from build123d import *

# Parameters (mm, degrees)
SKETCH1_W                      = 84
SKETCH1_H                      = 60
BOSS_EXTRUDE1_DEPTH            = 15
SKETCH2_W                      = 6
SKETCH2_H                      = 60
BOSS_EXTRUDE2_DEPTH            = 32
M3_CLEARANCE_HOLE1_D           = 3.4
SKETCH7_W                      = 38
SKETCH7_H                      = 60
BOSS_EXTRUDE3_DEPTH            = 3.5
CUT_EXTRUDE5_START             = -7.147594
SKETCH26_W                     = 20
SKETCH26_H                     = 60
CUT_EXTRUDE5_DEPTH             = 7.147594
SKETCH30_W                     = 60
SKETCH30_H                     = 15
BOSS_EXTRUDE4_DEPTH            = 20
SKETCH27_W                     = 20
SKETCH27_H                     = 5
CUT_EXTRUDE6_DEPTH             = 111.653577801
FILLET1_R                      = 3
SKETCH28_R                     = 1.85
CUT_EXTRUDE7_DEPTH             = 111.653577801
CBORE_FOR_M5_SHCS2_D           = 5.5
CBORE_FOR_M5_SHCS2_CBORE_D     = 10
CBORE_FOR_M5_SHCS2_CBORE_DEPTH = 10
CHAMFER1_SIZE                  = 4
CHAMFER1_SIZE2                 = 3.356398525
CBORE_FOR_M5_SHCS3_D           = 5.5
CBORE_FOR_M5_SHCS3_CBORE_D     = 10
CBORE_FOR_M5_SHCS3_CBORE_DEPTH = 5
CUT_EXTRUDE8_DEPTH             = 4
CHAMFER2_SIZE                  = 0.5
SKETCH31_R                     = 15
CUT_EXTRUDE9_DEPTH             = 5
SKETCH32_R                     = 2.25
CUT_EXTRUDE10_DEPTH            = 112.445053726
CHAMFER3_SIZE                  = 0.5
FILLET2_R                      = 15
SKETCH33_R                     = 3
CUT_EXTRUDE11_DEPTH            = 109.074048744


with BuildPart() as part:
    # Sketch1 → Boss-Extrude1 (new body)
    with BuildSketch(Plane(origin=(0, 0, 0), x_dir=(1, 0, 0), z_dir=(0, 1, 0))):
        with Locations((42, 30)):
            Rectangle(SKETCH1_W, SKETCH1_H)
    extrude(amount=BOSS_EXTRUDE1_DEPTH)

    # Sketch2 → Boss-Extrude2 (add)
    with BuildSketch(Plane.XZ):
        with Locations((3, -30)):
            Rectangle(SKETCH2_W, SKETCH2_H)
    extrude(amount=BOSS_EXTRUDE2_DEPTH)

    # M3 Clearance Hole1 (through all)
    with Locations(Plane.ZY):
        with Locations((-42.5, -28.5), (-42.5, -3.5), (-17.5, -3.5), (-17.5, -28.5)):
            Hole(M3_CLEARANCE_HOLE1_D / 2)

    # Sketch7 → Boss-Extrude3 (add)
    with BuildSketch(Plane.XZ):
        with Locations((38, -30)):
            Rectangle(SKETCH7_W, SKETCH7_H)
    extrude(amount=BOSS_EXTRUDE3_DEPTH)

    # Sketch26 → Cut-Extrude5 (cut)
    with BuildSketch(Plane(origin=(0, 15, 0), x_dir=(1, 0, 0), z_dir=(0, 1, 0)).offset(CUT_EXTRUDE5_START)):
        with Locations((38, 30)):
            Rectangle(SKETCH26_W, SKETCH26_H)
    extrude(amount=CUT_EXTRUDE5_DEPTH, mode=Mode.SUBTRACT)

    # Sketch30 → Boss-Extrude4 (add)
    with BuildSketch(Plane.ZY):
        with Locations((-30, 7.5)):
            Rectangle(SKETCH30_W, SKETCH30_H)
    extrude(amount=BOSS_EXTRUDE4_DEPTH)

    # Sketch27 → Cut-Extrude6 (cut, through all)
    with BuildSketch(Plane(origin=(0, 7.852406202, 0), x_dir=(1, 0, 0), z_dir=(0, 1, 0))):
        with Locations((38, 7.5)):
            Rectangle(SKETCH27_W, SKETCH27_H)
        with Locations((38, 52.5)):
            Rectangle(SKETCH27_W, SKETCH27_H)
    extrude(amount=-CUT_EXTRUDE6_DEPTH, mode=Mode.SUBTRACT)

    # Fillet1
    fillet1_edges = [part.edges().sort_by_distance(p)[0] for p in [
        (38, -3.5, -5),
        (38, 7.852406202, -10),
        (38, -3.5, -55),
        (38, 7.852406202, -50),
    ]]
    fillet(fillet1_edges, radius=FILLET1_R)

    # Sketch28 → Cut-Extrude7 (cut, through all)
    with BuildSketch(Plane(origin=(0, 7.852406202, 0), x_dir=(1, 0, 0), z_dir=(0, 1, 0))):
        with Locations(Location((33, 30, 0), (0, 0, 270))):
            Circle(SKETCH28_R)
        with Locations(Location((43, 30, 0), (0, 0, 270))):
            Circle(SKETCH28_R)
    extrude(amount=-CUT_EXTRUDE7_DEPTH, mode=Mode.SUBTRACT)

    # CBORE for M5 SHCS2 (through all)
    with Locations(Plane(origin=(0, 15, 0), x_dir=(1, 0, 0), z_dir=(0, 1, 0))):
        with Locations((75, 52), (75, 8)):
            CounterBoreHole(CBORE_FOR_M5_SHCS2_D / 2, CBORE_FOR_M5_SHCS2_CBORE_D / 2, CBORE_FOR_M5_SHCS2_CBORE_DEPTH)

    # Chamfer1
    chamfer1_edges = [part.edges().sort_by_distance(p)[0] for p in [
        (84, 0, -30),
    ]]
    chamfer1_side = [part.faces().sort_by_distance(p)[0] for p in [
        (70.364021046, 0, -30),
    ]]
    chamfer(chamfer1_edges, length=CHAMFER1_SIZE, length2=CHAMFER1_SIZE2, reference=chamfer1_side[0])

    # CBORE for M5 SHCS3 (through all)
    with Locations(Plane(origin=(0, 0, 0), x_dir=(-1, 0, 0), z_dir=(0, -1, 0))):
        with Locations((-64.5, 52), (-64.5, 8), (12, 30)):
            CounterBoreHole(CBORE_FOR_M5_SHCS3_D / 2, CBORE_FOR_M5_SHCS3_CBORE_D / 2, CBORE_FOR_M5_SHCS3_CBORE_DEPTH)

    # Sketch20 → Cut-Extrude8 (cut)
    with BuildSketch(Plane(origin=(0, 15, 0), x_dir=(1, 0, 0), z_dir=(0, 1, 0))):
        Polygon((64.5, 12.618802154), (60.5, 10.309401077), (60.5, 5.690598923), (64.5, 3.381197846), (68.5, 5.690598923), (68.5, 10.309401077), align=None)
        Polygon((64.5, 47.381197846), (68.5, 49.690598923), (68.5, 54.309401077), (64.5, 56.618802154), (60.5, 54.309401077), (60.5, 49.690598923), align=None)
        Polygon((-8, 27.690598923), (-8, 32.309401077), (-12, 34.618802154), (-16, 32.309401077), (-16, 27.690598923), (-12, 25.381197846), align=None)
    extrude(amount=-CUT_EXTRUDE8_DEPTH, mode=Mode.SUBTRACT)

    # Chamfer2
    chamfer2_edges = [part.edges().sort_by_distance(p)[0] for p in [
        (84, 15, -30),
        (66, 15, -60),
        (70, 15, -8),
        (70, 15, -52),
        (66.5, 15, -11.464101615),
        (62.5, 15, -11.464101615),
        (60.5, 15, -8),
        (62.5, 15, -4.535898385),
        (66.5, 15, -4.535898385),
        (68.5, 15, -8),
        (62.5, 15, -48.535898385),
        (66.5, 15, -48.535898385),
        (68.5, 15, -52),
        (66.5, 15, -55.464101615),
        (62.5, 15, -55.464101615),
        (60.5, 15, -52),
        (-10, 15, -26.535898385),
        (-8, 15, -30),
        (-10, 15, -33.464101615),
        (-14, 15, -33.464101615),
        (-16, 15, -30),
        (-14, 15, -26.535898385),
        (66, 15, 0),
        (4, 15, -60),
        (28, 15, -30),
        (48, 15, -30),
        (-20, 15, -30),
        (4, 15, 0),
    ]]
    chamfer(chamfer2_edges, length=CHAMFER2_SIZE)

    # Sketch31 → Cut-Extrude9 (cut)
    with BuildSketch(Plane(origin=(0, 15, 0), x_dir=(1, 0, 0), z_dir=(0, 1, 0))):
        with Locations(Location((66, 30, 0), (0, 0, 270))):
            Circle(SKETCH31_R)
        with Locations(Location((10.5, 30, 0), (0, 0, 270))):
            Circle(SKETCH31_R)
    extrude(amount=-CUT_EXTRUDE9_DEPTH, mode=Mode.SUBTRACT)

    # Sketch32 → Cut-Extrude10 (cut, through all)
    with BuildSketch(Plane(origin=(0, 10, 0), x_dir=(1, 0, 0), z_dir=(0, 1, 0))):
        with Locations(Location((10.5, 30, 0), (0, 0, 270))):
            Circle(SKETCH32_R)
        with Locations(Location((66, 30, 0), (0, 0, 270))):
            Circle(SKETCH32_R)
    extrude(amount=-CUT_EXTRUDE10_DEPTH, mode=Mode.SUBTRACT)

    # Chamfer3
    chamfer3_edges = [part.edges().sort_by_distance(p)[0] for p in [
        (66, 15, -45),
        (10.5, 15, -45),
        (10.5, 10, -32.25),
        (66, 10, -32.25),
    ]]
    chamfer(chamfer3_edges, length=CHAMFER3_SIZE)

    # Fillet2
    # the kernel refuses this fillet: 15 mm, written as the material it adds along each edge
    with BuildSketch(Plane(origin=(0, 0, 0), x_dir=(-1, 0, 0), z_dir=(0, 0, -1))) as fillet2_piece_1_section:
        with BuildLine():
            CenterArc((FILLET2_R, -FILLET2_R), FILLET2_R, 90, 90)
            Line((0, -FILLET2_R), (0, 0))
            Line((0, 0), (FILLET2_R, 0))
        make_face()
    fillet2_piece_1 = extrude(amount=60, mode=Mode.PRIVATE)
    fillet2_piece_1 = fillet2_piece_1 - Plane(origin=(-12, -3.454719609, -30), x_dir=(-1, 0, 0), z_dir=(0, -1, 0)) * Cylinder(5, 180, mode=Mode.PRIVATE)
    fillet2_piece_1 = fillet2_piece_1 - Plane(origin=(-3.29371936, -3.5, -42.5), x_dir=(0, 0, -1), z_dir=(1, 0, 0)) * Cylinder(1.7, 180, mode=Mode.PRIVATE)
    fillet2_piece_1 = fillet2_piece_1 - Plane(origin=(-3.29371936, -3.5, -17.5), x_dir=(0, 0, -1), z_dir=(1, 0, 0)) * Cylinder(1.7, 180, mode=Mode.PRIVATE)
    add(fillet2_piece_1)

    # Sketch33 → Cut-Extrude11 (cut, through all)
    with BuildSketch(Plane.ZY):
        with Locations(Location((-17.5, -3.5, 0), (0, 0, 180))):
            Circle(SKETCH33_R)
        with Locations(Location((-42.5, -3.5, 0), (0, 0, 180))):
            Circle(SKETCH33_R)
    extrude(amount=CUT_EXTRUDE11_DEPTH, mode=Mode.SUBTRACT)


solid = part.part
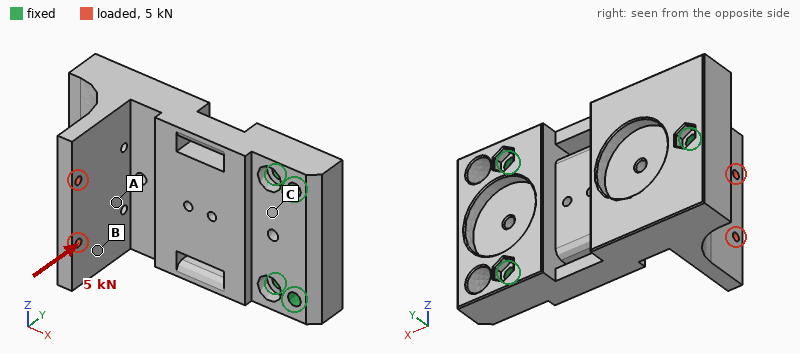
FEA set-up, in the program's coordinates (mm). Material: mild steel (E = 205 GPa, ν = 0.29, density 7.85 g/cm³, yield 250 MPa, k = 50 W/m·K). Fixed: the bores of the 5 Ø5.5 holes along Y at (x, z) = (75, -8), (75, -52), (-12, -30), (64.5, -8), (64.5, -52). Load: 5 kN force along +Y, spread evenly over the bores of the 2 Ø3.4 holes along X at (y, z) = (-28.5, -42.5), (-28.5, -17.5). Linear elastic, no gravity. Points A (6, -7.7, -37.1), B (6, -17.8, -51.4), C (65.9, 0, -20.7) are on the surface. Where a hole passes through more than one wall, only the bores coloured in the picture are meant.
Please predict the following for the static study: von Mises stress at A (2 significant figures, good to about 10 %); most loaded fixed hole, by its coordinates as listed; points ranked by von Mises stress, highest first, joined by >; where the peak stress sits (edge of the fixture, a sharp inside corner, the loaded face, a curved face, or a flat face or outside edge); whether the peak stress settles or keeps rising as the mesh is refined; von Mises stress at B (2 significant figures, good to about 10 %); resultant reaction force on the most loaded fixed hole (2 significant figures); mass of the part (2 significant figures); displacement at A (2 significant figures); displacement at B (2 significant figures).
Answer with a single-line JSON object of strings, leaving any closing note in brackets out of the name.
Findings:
{"von Mises stress at A": "25 MPa", "most loaded fixed hole, by its coordinates as listed": "(-12, -30)", "points ranked by von Mises stress, highest first, joined by >": "A > B > C", "where the peak stress sits": "edge of the fixture", "whether the peak stress settles or keeps rising as the mesh is refined": "keeps rising", "von Mises stress at B": "14 MPa", "resultant reaction force on the most loaded fixed hole": "4.2 kN", "mass of the part": "720 g", "displacement at A": "9.9 µm", "displacement at B": "12 µm"}
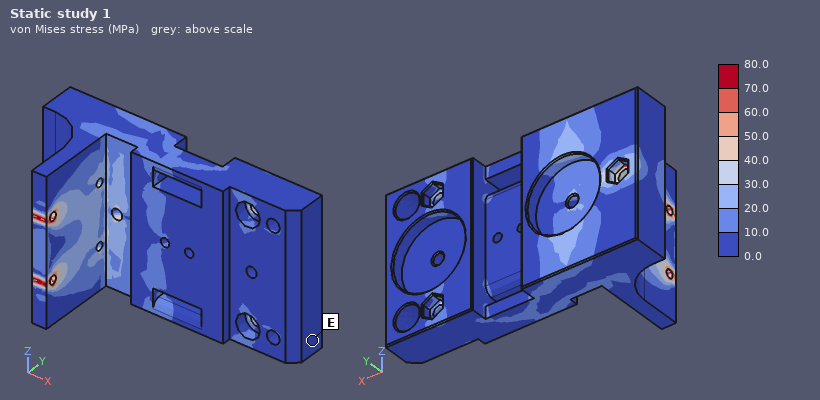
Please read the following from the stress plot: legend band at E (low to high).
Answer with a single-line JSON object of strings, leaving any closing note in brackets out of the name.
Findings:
{"legend band at E": "0.0 to 10.0 MPa"}
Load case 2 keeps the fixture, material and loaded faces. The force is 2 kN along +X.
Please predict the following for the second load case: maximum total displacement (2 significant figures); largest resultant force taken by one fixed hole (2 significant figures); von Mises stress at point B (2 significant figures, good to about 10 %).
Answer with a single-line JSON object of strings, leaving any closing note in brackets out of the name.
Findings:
{"maximum total displacement": "64 µm", "largest resultant force taken by one fixed hole": "1.2 kN", "von Mises stress at point B": "59 MPa"}
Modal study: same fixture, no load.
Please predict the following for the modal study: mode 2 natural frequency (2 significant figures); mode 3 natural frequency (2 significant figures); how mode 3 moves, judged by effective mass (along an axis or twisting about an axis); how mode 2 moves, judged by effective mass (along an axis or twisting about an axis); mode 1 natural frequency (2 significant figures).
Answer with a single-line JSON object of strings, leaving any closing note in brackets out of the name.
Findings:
{"mode 2 natural frequency": "4900 Hz", "mode 3 natural frequency": "7500 Hz", "how mode 3 moves, judged by effective mass": "along Y", "how mode 2 moves, judged by effective mass": "along Y", "mode 1 natural frequency": "3600 Hz"}
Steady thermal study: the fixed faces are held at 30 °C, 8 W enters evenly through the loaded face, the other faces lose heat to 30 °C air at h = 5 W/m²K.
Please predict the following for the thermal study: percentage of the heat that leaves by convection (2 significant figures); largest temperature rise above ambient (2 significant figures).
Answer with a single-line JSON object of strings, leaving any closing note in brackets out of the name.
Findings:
{"percentage of the heat that leaves by convection": "6.1 %", "largest temperature rise above ambient": "21 K"}
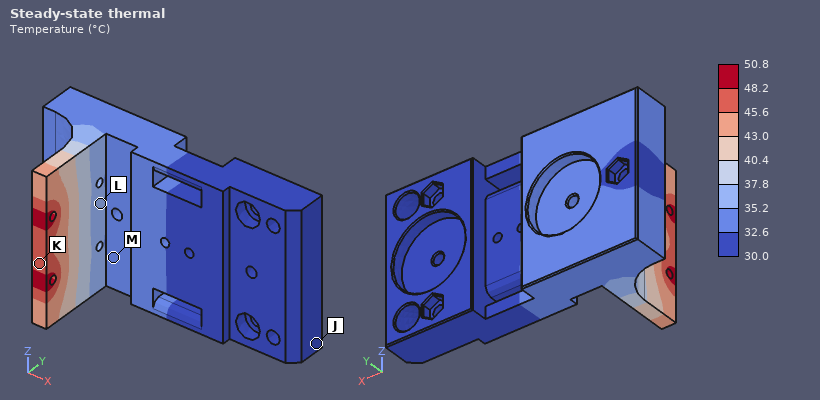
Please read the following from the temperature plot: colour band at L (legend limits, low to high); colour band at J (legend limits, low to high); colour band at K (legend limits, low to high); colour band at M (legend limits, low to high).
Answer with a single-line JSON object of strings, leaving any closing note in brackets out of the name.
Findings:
{"colour band at L": "35.2 to 37.8 °C", "colour band at J": "30.0 to 32.6 °C", "colour band at K": "45.6 to 48.2 °C", "colour band at M": "32.6 to 35.2 °C"}
